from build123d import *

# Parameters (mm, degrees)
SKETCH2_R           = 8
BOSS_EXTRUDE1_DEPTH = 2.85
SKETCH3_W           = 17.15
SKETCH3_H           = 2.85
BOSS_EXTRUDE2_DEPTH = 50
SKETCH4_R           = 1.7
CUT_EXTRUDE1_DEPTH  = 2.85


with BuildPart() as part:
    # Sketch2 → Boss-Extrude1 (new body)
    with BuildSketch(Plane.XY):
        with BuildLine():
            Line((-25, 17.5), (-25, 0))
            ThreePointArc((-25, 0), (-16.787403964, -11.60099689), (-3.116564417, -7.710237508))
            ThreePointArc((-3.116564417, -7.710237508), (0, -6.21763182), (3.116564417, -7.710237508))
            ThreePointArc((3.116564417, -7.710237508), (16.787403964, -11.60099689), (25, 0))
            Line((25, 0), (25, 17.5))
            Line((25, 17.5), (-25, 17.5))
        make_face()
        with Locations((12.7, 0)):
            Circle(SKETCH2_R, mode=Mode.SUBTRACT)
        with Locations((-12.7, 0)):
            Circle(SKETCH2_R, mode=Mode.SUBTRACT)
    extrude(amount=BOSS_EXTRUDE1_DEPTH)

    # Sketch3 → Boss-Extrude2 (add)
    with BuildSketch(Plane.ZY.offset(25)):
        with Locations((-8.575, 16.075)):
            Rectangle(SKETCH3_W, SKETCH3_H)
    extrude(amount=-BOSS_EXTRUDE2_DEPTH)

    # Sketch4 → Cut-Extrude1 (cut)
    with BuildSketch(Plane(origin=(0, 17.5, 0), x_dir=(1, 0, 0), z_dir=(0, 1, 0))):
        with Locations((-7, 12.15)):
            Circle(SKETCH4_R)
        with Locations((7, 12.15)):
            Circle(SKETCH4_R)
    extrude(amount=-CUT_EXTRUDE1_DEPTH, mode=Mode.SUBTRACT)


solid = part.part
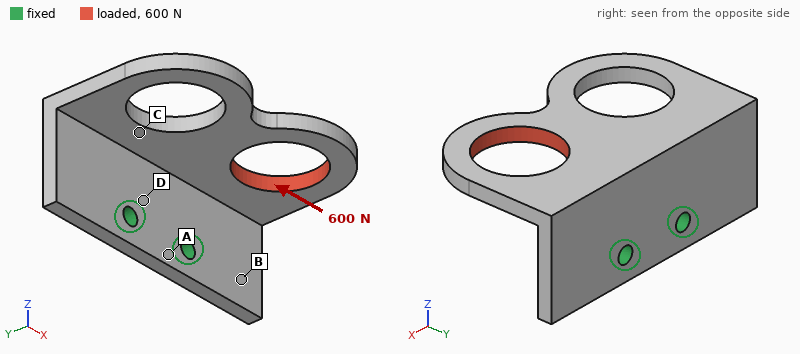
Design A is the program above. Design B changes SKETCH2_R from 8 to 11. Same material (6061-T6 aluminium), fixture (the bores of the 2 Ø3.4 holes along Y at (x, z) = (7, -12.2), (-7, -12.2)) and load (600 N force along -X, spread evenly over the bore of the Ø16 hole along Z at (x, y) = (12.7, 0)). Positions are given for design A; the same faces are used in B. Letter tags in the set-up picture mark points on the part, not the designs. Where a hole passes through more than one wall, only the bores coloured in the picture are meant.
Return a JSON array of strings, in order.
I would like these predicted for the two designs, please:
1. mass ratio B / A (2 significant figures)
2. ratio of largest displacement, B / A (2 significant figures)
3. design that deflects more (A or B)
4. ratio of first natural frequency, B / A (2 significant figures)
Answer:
["0.80", "1.9", "B", "1.3"]
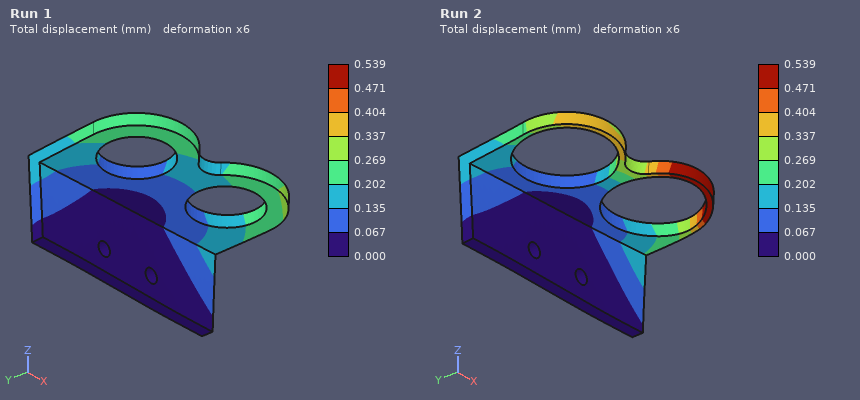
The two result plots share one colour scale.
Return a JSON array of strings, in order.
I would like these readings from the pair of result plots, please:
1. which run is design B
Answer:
["Run 2"]
